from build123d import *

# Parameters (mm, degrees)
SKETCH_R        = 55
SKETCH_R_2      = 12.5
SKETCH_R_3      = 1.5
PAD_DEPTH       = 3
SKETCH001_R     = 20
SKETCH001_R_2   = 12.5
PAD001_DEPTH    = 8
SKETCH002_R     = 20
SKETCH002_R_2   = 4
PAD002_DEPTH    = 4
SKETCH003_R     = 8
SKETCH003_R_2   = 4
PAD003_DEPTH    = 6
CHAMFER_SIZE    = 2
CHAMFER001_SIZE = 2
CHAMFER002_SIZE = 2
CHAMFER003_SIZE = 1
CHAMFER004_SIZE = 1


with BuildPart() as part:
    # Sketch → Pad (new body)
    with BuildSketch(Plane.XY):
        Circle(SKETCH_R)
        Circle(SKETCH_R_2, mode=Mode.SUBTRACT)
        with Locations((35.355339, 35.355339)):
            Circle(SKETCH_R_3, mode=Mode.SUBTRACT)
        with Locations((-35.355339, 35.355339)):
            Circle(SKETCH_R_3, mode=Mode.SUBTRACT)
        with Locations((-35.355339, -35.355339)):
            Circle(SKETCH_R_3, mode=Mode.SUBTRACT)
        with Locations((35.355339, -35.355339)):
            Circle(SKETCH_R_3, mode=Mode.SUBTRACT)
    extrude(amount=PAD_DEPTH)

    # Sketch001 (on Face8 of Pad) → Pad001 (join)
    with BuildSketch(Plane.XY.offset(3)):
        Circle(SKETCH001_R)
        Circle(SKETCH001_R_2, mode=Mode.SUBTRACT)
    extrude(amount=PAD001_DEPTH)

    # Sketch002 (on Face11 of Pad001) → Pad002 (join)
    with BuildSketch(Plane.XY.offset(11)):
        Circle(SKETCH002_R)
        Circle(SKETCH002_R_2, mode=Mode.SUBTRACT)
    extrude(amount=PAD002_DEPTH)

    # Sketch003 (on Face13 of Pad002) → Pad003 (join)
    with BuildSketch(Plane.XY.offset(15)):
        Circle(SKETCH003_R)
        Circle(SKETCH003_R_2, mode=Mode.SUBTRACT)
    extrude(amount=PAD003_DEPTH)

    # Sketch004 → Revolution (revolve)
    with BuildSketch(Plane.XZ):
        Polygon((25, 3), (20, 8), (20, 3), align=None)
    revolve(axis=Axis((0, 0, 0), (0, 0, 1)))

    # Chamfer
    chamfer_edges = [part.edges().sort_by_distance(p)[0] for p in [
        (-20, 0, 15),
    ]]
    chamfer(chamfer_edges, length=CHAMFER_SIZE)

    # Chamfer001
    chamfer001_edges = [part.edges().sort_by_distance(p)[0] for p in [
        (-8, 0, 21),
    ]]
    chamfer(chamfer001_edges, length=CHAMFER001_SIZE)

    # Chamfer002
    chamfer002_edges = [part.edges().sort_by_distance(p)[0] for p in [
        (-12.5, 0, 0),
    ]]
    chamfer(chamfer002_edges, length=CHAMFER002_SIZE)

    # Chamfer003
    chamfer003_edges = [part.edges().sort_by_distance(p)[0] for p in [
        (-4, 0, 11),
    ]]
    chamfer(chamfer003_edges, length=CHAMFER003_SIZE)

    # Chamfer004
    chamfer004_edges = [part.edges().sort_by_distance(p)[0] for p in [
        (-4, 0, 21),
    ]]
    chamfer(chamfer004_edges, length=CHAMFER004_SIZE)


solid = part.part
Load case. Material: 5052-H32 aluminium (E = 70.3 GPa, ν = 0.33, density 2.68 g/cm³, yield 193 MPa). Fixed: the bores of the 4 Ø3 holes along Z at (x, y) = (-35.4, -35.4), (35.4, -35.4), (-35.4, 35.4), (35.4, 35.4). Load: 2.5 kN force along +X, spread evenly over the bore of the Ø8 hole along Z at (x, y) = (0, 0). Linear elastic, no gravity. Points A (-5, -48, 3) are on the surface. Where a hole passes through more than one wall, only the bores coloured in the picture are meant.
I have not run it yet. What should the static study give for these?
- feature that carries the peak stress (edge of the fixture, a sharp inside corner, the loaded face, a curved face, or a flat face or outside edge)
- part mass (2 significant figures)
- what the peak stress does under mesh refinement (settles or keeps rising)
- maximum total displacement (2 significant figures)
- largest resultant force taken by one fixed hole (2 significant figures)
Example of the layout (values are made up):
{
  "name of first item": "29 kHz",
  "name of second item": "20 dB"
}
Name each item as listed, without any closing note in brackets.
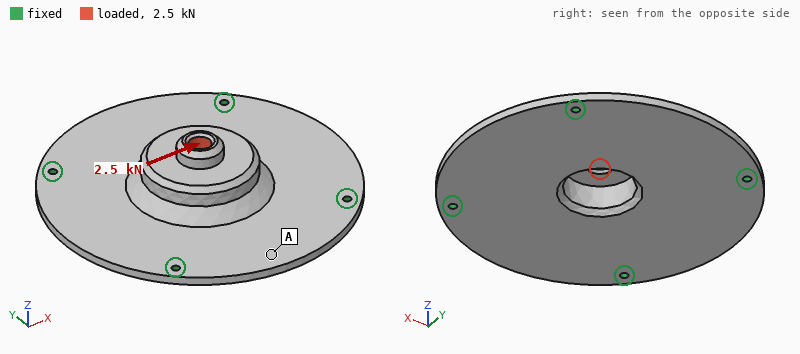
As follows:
{
  "feature that carries the peak stress": "edge of the fixture",
  "part mass": "110 g",
  "what the peak stress does under mesh refinement": "keeps rising",
  "maximum total displacement": "0.10 mm",
  "largest resultant force taken by one fixed hole": "720 N"
}
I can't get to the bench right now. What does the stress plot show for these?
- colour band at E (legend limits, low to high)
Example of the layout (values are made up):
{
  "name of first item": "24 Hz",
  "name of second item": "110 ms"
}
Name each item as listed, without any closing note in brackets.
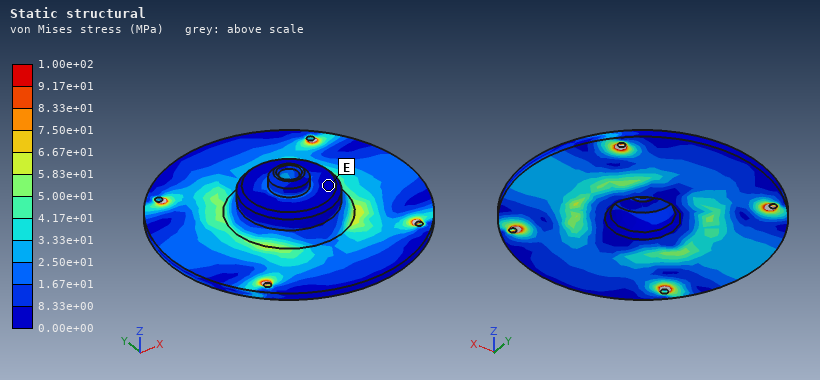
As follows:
{
  "colour band at E": "0.00e+00 to 8.33e+00 MPa"
}
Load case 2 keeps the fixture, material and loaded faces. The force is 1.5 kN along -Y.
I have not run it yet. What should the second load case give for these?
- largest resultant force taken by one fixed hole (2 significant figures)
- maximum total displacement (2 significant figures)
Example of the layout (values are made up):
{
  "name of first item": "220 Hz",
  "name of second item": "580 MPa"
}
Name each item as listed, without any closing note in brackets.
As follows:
{
  "largest resultant force taken by one fixed hole": "430 N",
  "maximum total displacement": "62 µm"
}
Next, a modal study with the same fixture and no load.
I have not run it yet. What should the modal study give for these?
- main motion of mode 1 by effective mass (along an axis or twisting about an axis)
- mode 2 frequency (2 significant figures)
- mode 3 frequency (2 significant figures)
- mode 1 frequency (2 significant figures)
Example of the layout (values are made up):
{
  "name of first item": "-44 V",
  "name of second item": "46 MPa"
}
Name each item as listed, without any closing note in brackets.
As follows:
{
  "main motion of mode 1 by effective mass": "along Z",
  "mode 2 frequency": "2800 Hz",
  "mode 3 frequency": "2800 Hz",
  "mode 1 frequency": "2000 Hz"
}
